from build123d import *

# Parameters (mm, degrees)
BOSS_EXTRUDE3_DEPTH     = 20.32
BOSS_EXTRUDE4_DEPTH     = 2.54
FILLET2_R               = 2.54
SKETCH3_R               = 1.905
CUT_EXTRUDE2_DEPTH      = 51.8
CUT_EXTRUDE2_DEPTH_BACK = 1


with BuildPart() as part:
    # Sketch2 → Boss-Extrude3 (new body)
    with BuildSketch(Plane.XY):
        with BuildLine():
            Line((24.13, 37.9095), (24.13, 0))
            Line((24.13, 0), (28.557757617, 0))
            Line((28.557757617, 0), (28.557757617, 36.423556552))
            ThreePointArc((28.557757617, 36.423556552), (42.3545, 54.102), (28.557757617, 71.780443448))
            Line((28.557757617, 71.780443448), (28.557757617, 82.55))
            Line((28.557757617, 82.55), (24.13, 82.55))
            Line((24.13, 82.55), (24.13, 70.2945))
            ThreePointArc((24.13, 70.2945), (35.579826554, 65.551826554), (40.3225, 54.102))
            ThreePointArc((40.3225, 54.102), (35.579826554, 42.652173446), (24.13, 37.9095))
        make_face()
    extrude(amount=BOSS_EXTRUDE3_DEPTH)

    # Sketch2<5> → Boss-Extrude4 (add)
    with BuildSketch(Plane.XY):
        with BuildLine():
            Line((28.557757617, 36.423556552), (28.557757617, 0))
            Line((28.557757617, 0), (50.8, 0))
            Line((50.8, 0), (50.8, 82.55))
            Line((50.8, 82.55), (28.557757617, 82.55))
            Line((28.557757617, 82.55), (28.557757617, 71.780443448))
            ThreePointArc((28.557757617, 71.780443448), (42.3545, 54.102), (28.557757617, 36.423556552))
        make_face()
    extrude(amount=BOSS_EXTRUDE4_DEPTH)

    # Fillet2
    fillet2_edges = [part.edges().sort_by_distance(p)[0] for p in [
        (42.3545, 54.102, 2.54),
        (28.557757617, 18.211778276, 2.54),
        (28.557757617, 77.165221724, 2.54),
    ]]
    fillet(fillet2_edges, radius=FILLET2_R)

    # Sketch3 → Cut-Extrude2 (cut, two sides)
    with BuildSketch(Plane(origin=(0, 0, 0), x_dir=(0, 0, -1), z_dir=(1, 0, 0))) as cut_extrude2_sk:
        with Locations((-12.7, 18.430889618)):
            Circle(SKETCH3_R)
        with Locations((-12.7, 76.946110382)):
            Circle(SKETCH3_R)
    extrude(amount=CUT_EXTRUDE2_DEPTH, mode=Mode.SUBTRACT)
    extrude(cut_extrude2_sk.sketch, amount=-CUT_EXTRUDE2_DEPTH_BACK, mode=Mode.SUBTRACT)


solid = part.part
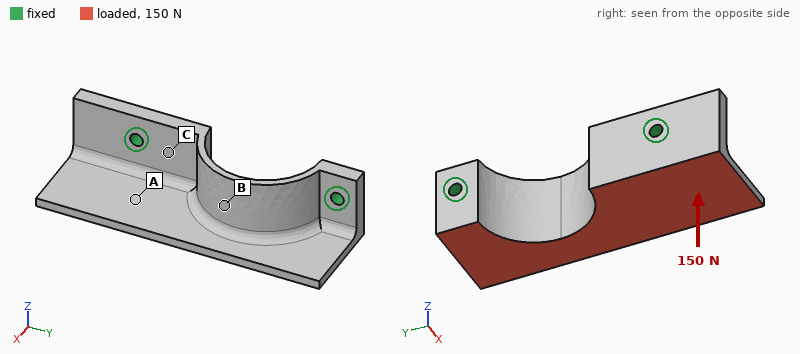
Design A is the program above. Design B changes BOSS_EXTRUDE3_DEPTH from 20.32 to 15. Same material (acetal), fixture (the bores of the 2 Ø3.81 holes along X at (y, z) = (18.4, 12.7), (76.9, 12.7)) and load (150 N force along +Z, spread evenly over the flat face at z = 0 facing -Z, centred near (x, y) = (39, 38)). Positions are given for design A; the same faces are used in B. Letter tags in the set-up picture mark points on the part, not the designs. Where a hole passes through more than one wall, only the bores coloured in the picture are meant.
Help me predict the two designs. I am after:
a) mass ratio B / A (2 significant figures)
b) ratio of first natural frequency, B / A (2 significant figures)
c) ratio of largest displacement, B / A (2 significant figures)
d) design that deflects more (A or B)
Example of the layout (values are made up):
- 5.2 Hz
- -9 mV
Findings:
- 0.84
- 0.89
- 1.2
- B
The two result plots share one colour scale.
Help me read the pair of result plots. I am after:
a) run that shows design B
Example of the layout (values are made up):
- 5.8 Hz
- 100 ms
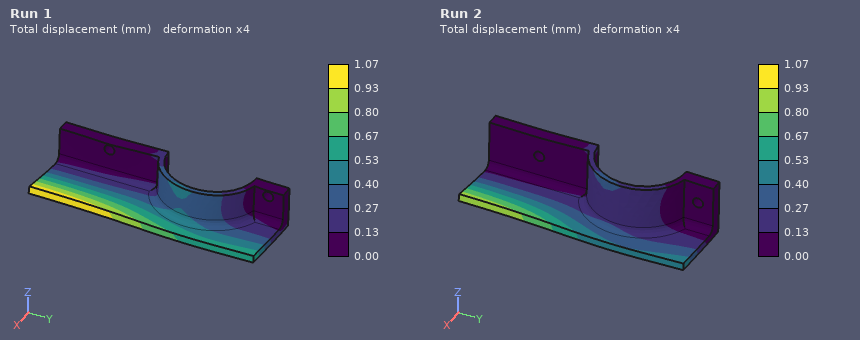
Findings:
- Run 1
